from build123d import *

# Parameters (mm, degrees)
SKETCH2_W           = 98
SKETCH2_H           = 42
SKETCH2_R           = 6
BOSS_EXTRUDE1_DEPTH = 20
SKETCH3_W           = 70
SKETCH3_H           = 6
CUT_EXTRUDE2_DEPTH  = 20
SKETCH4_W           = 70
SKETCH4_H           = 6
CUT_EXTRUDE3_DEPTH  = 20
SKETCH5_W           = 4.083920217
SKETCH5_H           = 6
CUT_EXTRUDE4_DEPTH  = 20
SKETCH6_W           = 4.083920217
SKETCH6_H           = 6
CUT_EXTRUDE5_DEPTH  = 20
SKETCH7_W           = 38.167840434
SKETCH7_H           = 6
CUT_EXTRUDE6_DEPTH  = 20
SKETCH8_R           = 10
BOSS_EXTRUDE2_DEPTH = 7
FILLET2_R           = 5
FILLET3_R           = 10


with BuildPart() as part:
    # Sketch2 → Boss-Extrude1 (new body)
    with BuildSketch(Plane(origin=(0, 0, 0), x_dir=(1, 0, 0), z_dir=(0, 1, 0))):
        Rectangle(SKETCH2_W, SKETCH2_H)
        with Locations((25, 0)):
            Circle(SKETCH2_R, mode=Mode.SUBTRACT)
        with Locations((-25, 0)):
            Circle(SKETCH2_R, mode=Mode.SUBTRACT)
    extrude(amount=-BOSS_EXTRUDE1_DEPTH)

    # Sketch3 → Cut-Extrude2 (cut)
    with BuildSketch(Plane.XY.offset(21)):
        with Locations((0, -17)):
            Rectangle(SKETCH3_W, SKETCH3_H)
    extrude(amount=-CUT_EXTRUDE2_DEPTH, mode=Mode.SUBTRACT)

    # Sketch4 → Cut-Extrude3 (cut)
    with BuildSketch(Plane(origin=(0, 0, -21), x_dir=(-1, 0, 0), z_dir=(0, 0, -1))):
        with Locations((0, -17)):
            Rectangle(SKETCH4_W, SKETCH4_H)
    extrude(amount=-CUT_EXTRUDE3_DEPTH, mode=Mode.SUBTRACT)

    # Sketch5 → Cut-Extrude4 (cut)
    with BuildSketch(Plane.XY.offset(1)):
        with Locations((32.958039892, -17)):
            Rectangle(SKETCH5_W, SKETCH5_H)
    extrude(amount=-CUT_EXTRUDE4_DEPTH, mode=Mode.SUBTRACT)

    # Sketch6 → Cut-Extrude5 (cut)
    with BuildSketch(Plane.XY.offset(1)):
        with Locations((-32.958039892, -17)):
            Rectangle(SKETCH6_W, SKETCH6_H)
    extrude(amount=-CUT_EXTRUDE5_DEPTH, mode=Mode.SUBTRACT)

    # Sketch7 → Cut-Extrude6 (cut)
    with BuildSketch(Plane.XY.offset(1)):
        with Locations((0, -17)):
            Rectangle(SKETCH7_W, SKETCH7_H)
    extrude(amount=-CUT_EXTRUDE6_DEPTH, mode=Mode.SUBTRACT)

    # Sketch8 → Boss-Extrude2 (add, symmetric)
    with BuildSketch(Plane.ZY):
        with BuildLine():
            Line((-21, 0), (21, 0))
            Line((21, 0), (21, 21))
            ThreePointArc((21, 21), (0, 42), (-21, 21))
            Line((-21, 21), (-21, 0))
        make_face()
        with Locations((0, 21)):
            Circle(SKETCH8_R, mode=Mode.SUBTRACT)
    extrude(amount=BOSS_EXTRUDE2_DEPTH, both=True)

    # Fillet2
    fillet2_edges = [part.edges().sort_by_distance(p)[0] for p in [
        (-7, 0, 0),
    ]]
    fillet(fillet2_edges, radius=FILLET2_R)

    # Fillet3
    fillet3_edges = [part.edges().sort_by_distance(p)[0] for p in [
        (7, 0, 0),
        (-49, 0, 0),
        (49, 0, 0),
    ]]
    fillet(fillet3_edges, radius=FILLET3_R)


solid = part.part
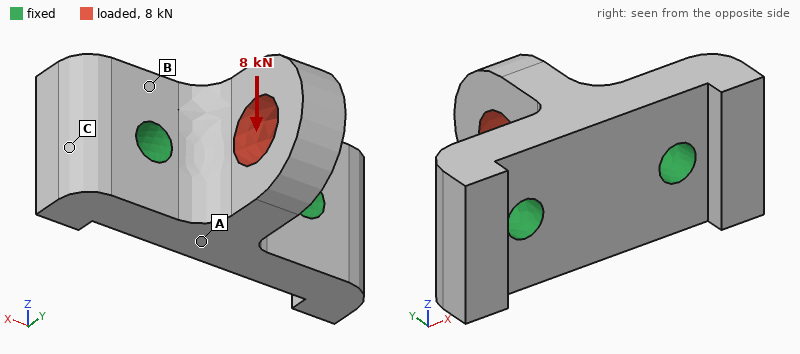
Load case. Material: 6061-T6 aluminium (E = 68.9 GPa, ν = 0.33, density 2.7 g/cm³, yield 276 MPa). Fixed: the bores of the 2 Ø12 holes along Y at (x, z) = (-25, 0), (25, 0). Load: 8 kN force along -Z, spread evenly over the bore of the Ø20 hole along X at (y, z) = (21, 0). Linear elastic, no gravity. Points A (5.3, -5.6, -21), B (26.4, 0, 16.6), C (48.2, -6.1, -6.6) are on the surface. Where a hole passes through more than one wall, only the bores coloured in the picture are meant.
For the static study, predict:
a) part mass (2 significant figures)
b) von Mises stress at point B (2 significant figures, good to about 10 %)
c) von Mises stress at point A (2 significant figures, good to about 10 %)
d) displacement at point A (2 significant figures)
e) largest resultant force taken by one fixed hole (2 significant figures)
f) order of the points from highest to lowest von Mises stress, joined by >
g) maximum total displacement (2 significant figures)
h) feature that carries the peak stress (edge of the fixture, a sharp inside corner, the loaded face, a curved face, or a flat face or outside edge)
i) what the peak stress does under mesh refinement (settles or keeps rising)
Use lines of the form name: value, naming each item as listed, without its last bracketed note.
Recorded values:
part mass: 210 g
von Mises stress at point B: 21 MPa
von Mises stress at point A: 34 MPa
displacement at point A: 0.037 mm
largest resultant force taken by one fixed hole: 4.1 kN
order of the points from highest to lowest von Mises stress, joined by >: A > B > C
maximum total displacement: 0.14 mm
feature that carries the peak stress: edge of the fixture
what the peak stress does under mesh refinement: keeps rising
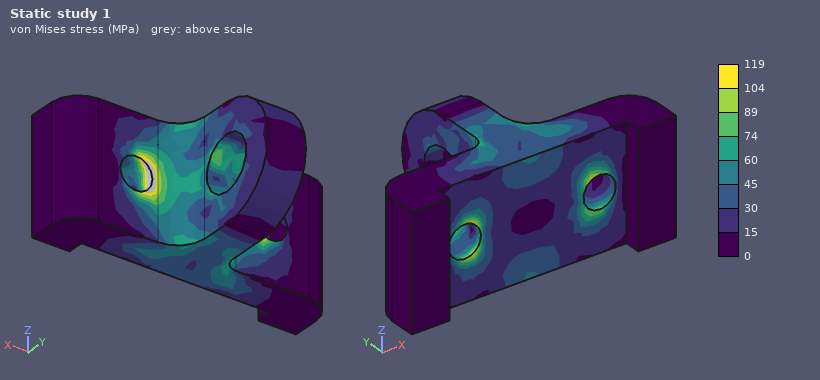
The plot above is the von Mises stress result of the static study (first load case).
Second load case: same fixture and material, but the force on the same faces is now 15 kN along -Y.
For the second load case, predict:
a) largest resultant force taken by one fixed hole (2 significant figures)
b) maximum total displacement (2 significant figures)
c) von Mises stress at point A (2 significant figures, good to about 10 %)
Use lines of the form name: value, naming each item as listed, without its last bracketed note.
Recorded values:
largest resultant force taken by one fixed hole: 7.9 kN
maximum total displacement: 44 µm
von Mises stress at point A: 11 MPa
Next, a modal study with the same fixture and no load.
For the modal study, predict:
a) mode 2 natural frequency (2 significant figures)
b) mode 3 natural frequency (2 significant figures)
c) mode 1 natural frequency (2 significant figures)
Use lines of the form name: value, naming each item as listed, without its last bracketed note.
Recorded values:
mode 2 natural frequency: 6500 Hz
mode 3 natural frequency: 13 kHz
mode 1 natural frequency: 6300 Hz
